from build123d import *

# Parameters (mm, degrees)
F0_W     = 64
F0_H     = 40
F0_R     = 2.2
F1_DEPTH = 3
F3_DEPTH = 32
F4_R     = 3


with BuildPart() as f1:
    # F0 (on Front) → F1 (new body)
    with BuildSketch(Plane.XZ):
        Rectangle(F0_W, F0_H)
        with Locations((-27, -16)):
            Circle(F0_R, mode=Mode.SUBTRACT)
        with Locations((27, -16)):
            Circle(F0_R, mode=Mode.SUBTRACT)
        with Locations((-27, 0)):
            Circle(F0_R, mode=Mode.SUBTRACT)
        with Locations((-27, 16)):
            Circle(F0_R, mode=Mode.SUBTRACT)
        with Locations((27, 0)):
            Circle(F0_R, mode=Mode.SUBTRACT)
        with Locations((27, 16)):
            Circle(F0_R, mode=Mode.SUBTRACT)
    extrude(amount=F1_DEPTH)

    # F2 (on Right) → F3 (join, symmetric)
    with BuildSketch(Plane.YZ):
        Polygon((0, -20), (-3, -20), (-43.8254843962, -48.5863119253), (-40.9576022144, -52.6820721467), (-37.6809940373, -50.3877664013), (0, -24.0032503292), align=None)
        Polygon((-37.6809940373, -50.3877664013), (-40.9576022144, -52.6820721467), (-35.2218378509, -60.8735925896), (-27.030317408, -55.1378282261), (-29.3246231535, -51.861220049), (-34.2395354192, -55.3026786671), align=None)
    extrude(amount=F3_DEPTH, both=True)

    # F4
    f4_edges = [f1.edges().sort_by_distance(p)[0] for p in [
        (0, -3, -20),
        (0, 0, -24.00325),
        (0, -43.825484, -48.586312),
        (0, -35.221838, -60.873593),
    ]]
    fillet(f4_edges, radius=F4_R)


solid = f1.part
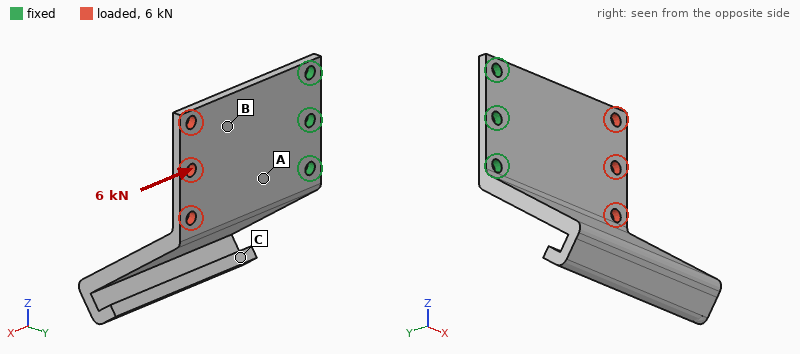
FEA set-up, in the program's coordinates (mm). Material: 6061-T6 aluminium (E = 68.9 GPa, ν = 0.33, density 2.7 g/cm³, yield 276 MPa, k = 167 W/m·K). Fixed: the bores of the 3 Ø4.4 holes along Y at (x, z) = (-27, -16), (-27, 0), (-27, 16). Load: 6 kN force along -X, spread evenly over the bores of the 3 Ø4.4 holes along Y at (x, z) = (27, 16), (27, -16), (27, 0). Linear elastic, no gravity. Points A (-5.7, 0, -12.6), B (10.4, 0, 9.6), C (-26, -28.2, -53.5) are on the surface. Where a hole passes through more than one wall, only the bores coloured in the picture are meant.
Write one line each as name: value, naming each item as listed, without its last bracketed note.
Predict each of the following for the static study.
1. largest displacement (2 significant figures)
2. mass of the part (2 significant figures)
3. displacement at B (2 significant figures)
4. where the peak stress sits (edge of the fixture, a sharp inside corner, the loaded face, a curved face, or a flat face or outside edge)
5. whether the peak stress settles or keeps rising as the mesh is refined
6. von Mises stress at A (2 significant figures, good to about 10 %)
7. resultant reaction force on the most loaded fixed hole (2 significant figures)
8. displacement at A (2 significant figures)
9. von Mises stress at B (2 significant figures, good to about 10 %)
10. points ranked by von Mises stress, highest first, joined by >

largest displacement: 60 µm
mass of the part: 75 g
displacement at B: 30 µm
where the peak stress sits: a sharp inside corner
whether the peak stress settles or keeps rising as the mesh is refined: keeps rising
von Mises stress at A: 31 MPa
resultant reaction force on the most loaded fixed hole: 2.1 kN
displacement at A: 11 µm
von Mises stress at B: 50 MPa
points ranked by von Mises stress, highest first, joined by >: B > A > C
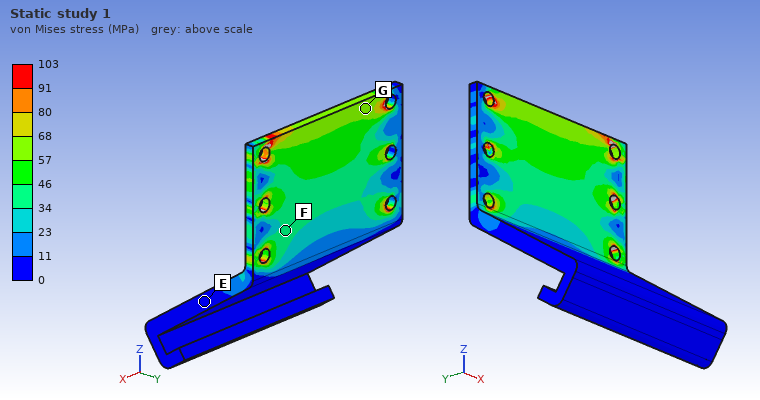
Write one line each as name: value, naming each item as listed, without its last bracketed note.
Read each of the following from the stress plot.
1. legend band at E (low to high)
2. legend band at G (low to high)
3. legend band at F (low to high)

legend band at E: 0 to 11 MPa
legend band at G: 57 to 68 MPa
legend band at F: 34 to 46 MPa
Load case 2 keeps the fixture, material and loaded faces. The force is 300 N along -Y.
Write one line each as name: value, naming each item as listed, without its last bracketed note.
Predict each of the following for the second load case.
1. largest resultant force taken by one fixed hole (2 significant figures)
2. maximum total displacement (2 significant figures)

largest resultant force taken by one fixed hole: 270 N
maximum total displacement: 1.0 mm
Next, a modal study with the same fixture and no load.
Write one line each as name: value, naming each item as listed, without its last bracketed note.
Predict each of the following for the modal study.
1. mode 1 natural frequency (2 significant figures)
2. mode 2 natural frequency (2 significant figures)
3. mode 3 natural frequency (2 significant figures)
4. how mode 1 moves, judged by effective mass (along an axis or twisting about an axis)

mode 1 natural frequency: 420 Hz
mode 2 natural frequency: 730 Hz
mode 3 natural frequency: 1900 Hz
how mode 1 moves, judged by effective mass: along Y
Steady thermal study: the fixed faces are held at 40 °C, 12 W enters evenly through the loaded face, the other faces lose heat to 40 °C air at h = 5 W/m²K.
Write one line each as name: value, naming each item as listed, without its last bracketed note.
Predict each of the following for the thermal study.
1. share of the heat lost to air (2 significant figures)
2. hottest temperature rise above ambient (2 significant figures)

share of the heat lost to air: 5.7 %
hottest temperature rise above ambient: 26 K
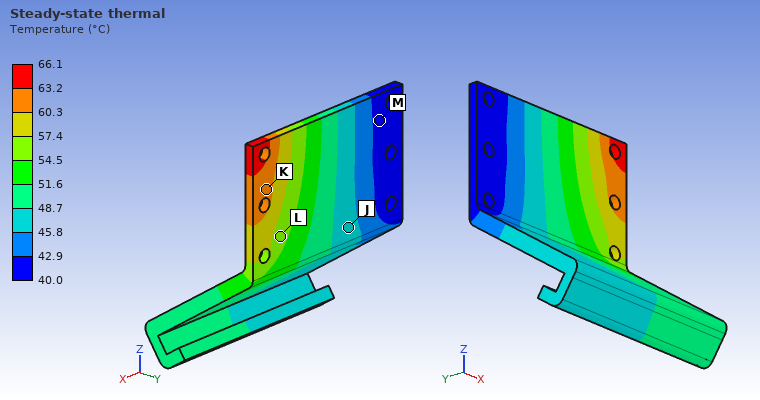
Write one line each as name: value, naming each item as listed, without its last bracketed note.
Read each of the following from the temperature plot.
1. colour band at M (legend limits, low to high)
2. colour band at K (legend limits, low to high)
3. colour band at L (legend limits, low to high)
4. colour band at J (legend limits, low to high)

colour band at M: 40.0 to 42.9 °C
colour band at K: 60.3 to 63.2 °C
colour band at L: 54.5 to 57.4 °C
colour band at J: 45.8 to 48.7 °C
